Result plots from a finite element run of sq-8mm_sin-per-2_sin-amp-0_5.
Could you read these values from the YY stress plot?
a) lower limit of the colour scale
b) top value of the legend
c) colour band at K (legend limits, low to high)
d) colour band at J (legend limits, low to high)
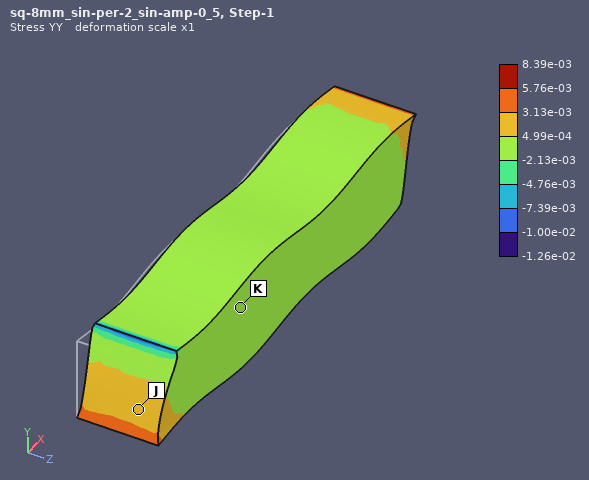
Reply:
-1.26e-02
8.39e-03
-2.13e-03 to 4.99e-04
4.99e-04 to 3.13e-03
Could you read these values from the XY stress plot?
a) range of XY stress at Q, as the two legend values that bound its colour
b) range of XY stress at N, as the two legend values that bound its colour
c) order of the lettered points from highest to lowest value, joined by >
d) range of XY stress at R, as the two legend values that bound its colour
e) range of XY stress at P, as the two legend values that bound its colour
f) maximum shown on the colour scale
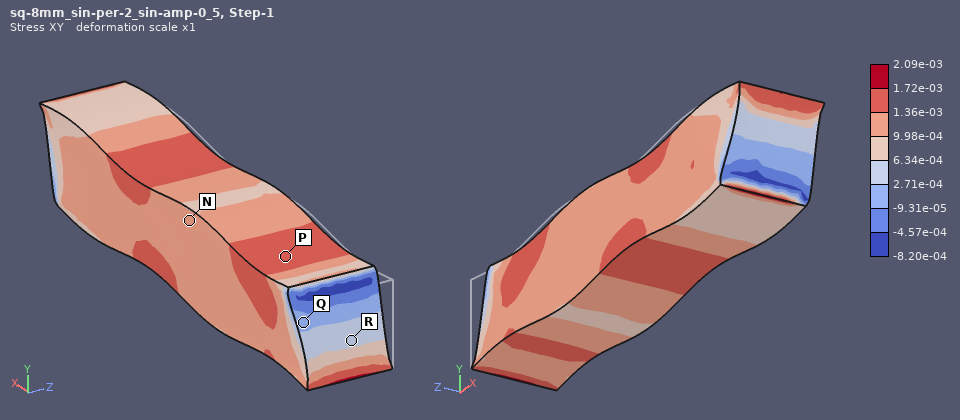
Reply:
-9.31e-05 to 2.71e-04
9.98e-04 to 1.36e-03
P > N > R > Q
2.71e-04 to 6.34e-04
1.36e-03 to 1.72e-03
2.09e-03
